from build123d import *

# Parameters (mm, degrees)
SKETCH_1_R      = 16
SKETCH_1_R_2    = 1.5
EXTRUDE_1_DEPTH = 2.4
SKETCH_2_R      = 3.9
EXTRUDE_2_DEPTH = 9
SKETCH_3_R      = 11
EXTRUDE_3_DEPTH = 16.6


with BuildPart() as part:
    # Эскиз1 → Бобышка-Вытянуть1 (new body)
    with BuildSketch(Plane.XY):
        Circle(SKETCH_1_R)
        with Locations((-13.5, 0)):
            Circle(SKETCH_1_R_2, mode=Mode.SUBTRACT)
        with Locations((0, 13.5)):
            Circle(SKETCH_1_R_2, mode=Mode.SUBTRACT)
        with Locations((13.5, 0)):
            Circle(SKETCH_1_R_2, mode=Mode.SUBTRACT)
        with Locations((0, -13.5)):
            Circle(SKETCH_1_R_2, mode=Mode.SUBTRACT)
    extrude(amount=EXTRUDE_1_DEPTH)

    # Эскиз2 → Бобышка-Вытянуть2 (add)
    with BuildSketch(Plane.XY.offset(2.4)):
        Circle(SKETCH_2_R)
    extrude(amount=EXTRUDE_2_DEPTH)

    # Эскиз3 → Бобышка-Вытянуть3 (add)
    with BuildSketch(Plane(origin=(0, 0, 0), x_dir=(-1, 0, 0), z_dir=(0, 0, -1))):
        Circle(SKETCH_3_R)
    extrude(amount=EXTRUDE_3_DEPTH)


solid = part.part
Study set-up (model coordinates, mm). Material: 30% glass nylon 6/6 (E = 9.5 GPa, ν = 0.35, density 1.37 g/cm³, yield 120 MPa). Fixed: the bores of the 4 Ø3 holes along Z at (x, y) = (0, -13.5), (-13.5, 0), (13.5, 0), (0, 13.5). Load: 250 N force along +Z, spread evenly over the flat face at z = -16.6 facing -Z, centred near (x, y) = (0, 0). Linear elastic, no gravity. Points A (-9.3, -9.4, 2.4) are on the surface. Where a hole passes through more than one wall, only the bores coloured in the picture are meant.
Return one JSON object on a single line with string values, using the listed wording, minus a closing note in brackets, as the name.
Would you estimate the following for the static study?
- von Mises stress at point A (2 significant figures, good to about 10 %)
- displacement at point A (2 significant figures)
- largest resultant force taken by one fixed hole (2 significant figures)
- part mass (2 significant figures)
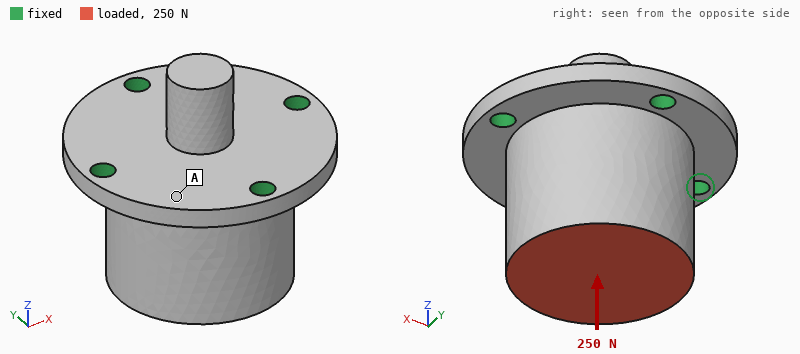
{"von Mises stress at point A": "1.7 MPa", "displacement at point A": "4.7 µm", "largest resultant force taken by one fixed hole": "67 N", "part mass": "12 g"}
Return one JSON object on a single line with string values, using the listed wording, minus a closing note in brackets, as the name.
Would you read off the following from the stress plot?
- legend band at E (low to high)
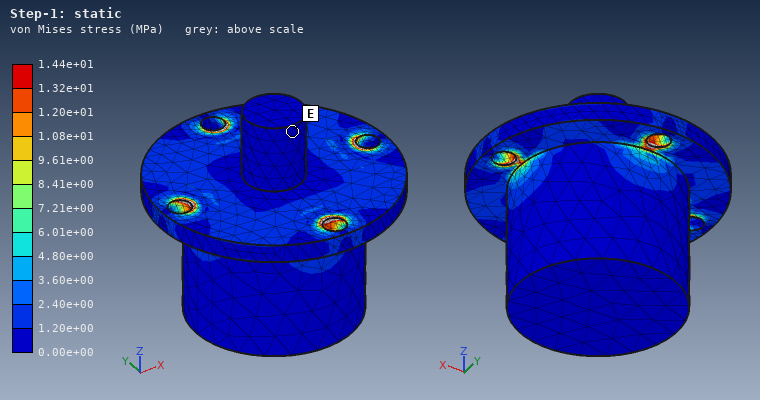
{"legend band at E": "0.00e+00 to 1.20e+00 MPa"}
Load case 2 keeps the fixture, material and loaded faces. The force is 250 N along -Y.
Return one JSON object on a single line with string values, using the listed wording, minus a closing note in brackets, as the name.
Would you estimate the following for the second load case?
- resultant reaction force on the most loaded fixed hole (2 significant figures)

{"resultant reaction force on the most loaded fixed hole": "210 N"}
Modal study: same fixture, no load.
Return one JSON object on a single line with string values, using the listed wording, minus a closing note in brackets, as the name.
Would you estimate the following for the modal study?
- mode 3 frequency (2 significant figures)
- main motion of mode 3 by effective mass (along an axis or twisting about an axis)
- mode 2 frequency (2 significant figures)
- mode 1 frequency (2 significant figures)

{"mode 3 frequency": "10 kHz", "main motion of mode 3 by effective mass": "along Z", "mode 2 frequency": "7600 Hz", "mode 1 frequency": "7500 Hz"}
